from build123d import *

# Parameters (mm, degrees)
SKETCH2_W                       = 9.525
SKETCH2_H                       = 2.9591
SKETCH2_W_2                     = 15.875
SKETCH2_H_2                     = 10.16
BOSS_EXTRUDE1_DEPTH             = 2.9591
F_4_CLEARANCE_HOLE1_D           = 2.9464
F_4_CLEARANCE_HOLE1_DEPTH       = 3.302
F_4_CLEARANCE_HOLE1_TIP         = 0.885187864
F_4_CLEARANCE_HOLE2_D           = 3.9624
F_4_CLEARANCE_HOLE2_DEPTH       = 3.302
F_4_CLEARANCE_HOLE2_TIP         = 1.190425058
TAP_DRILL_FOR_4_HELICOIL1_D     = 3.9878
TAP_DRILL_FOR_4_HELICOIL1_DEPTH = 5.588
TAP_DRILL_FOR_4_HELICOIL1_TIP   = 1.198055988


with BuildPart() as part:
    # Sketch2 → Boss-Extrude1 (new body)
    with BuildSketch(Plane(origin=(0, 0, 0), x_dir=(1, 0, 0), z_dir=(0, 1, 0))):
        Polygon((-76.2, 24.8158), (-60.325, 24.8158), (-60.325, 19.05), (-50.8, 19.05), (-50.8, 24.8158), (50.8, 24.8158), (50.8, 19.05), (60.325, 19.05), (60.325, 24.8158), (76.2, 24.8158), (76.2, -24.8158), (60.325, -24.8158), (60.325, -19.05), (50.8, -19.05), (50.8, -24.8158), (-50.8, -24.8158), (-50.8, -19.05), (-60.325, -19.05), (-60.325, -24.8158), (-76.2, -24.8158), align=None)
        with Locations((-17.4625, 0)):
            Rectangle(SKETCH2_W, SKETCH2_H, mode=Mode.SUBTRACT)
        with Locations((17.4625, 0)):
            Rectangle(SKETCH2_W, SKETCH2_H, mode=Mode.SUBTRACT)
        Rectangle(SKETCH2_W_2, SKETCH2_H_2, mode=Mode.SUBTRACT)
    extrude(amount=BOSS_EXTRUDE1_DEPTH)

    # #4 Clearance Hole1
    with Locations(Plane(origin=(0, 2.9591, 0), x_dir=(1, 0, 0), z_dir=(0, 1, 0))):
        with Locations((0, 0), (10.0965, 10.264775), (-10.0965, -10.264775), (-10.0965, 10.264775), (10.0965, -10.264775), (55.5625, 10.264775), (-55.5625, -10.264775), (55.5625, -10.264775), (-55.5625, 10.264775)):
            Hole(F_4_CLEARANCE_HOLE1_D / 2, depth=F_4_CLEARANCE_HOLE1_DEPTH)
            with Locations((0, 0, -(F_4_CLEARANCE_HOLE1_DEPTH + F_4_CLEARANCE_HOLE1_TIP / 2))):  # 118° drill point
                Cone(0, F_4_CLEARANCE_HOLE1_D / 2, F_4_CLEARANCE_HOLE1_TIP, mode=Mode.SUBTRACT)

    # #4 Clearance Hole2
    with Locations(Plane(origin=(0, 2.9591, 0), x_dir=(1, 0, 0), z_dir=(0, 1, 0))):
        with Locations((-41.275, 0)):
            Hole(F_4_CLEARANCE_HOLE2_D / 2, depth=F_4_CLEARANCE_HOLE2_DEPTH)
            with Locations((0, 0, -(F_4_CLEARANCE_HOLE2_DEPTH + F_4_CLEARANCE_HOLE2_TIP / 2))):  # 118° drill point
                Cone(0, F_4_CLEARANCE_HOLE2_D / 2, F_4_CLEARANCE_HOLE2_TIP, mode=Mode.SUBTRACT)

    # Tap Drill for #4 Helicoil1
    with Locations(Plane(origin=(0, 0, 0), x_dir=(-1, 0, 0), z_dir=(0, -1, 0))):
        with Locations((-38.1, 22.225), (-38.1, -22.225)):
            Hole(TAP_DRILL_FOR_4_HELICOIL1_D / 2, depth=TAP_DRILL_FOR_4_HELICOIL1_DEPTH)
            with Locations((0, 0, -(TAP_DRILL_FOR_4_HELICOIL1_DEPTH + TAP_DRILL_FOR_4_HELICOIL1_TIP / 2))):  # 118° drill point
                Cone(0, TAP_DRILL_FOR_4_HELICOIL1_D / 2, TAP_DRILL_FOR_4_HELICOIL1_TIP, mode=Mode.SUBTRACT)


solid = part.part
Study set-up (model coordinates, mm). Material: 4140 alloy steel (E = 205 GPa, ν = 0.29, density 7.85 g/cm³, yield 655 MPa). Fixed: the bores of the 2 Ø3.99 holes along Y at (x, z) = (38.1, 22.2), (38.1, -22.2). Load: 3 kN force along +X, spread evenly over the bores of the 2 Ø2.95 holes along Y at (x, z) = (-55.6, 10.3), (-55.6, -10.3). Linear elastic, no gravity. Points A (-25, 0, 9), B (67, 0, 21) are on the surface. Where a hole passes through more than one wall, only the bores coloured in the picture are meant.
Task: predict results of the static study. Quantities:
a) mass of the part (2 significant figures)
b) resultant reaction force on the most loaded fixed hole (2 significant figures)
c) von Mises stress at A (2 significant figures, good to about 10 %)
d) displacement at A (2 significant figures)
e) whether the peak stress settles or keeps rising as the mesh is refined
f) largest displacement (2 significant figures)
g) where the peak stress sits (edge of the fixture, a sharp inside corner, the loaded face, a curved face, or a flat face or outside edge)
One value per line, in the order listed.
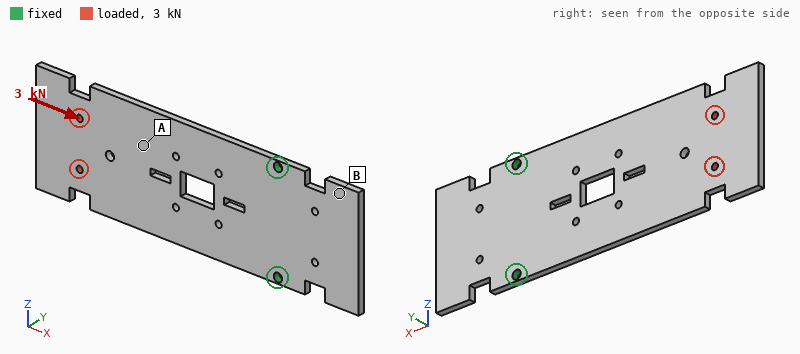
160 g
1.5 kN
22 MPa
8.8 µm
keeps rising
13 µm
edge of the fixture
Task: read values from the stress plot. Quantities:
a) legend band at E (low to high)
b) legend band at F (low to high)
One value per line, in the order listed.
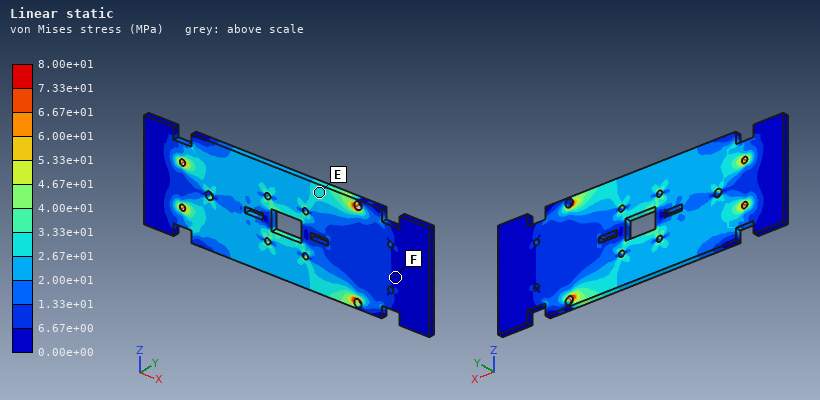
2.67e+01 to 3.33e+01 MPa
0.00e+00 to 6.67e+00 MPa
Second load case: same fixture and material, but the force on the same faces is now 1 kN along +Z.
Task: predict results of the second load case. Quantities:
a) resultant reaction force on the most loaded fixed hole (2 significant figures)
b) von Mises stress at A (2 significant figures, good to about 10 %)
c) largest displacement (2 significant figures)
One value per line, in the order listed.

2.2 kN
18 MPa
79 µm
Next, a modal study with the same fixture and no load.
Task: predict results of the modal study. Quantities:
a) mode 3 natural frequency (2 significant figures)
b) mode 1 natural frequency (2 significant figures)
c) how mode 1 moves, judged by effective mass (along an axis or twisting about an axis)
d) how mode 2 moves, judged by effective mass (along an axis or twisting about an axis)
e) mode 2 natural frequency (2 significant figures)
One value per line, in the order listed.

1100 Hz
180 Hz
along Y
twisting about X
900 Hz
